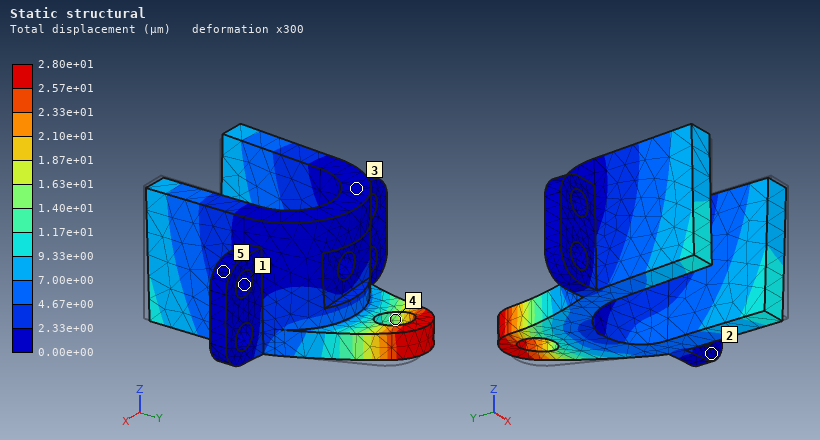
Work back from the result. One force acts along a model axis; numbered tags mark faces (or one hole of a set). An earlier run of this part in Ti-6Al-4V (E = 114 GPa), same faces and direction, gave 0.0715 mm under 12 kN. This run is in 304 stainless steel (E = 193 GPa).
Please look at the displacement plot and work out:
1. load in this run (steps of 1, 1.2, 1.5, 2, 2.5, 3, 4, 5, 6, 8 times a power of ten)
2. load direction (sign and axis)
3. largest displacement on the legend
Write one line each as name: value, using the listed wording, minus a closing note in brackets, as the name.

load in this run: 8 kN
load direction: -X
largest displacement on the legend: 2.80e+01 µm
